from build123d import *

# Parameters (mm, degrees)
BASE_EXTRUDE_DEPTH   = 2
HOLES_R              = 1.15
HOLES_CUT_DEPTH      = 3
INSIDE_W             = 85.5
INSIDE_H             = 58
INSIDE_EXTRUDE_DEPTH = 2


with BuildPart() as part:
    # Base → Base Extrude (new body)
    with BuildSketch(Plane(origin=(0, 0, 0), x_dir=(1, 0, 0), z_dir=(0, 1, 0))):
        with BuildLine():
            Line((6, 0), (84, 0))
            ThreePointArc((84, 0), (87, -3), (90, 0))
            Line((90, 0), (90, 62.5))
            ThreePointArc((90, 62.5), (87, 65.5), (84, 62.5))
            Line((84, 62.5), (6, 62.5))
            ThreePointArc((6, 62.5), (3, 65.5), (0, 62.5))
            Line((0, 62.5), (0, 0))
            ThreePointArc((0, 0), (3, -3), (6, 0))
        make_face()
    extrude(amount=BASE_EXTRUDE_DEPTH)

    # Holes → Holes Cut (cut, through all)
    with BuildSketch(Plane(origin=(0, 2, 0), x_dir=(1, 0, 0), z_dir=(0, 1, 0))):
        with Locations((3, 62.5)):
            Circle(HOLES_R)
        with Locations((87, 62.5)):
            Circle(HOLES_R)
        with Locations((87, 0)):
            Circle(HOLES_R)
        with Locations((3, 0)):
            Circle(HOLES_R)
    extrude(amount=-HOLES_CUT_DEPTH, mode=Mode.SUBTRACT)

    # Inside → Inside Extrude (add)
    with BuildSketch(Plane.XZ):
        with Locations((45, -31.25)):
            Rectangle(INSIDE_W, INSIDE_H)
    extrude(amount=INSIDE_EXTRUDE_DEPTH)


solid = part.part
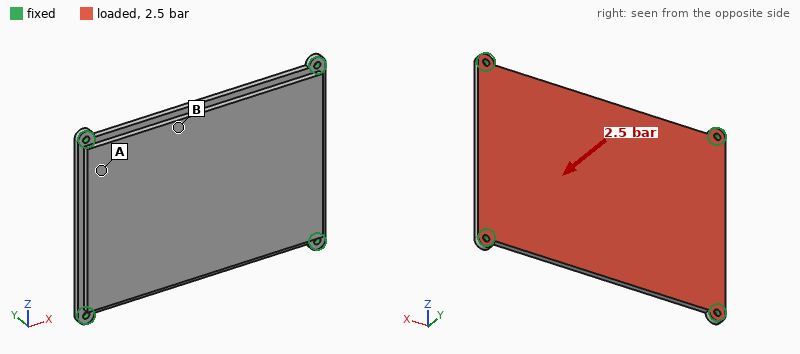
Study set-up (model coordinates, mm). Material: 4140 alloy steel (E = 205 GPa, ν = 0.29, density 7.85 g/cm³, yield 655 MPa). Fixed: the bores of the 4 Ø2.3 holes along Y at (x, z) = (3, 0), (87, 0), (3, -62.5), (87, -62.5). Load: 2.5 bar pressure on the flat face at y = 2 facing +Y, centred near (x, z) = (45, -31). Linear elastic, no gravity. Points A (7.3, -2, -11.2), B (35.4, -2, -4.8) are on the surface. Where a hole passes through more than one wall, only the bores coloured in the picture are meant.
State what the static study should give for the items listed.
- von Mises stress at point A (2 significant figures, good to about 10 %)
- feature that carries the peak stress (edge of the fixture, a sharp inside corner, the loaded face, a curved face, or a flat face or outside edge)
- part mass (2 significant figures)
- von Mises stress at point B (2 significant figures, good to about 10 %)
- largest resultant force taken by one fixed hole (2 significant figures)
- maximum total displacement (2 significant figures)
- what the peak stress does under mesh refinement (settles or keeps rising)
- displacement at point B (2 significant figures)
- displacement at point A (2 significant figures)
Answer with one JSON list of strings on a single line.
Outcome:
["38 MPa", "edge of the fixture", "170 g", "65 MPa", "920 N", "0.11 mm", "keeps rising", "0.097 mm", "0.030 mm"]
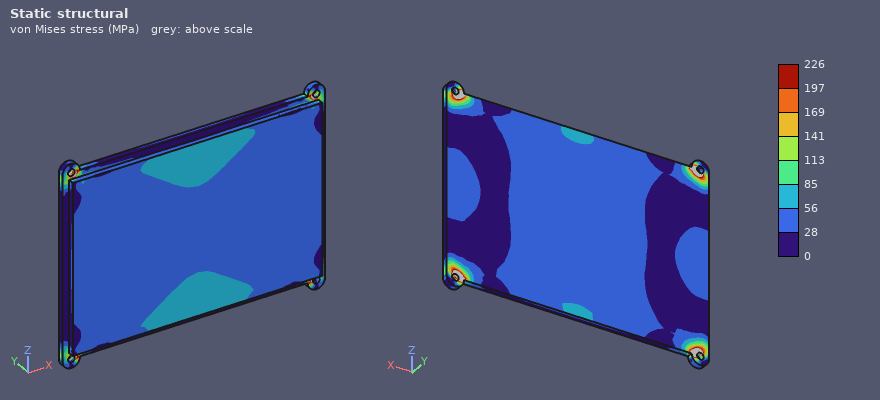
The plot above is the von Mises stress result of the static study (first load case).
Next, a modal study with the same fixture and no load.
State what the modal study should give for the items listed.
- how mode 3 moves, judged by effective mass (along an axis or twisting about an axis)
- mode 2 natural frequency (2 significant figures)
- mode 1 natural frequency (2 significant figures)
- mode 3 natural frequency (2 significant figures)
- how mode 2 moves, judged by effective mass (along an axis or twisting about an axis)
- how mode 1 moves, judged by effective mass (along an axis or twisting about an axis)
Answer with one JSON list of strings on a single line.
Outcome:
["twisting about Z", "3100 Hz", "1600 Hz", "3600 Hz", "twisting about X", "along Y"]
